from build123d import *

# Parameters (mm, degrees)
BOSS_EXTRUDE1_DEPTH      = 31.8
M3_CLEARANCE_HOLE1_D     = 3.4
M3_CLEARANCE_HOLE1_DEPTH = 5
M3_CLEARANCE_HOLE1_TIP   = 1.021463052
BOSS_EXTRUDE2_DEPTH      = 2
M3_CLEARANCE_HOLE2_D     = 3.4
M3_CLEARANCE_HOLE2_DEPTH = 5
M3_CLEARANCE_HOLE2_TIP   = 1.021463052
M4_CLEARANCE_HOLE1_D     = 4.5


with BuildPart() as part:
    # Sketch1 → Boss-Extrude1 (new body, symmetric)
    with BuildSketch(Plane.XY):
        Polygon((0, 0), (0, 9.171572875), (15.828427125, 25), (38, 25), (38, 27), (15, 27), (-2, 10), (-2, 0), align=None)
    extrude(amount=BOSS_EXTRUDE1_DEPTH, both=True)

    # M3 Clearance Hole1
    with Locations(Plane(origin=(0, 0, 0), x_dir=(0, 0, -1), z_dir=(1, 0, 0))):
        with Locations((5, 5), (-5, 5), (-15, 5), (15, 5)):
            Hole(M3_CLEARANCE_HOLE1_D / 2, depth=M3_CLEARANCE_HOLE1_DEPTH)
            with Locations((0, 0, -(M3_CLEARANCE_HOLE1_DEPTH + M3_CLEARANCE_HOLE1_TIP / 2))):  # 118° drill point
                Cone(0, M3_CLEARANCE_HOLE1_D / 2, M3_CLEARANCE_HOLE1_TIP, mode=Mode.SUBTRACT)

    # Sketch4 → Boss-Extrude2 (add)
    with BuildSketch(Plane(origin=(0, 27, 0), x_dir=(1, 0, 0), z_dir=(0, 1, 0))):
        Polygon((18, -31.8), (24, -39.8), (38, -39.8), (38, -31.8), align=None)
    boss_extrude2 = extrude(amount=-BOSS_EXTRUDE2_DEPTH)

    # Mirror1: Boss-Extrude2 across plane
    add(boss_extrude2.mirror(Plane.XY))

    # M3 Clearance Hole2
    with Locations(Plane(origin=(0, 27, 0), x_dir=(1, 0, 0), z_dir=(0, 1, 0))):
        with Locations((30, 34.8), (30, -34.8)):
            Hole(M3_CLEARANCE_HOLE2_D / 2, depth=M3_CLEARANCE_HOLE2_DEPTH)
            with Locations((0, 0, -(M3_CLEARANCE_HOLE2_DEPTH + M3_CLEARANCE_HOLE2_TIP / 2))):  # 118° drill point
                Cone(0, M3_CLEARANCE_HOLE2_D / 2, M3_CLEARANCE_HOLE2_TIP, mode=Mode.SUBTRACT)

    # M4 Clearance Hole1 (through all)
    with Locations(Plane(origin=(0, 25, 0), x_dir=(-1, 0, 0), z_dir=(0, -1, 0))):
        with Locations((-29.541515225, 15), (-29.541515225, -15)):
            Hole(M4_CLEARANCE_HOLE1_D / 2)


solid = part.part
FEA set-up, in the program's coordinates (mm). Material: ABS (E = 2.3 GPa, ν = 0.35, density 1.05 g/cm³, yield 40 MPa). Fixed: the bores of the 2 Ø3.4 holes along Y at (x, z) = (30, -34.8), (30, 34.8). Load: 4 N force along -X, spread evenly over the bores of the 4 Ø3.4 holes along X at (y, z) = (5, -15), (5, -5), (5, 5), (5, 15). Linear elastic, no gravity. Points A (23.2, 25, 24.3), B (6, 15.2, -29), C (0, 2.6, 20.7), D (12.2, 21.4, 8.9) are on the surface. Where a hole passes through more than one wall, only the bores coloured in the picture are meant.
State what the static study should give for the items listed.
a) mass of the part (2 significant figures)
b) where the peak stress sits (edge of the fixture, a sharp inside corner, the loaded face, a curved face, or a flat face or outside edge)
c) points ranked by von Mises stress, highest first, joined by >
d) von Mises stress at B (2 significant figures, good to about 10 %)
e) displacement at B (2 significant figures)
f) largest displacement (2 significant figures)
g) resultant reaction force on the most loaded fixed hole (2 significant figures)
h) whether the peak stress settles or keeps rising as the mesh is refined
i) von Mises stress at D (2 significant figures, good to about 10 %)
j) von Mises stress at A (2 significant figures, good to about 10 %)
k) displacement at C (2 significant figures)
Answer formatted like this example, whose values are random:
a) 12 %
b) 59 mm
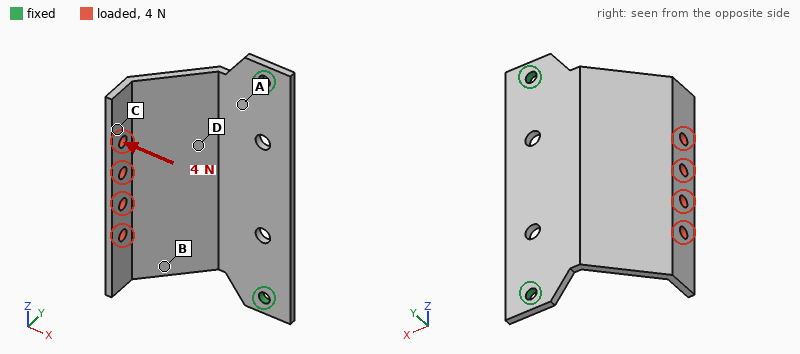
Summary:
a) 7.8 g
b) edge of the fixture
c) A > D > B > C
d) 0.87 MPa
e) 0.44 mm
f) 0.93 mm
g) 2.8 N
h) keeps rising
i) 1.4 MPa
j) 2.1 MPa
k) 0.82 mm
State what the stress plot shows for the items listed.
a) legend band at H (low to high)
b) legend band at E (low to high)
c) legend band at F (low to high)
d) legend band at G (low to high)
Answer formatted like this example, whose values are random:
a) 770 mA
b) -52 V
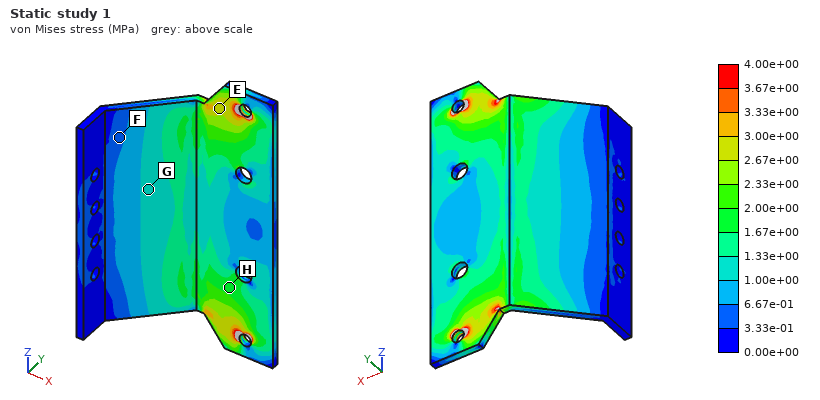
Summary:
a) 1.67e+00 to 2.00e+00 MPa
b) 2.67e+00 to 3.00e+00 MPa
c) 3.33e-01 to 6.67e-01 MPa
d) 1.00e+00 to 1.33e+00 MPa
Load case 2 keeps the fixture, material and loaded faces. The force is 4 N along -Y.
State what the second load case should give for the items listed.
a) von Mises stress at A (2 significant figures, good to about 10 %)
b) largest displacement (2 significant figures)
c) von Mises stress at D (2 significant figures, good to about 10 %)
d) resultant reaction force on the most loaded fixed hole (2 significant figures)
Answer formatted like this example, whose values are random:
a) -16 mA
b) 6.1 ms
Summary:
a) 2.3 MPa
b) 0.98 mm
c) 1.1 MPa
d) 2.3 N
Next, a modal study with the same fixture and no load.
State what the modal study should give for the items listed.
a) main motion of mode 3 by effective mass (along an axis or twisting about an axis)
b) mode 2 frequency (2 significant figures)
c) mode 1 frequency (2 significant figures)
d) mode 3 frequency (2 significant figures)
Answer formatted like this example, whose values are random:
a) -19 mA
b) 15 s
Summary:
a) along Y
b) 450 Hz
c) 190 Hz
d) 750 Hz
